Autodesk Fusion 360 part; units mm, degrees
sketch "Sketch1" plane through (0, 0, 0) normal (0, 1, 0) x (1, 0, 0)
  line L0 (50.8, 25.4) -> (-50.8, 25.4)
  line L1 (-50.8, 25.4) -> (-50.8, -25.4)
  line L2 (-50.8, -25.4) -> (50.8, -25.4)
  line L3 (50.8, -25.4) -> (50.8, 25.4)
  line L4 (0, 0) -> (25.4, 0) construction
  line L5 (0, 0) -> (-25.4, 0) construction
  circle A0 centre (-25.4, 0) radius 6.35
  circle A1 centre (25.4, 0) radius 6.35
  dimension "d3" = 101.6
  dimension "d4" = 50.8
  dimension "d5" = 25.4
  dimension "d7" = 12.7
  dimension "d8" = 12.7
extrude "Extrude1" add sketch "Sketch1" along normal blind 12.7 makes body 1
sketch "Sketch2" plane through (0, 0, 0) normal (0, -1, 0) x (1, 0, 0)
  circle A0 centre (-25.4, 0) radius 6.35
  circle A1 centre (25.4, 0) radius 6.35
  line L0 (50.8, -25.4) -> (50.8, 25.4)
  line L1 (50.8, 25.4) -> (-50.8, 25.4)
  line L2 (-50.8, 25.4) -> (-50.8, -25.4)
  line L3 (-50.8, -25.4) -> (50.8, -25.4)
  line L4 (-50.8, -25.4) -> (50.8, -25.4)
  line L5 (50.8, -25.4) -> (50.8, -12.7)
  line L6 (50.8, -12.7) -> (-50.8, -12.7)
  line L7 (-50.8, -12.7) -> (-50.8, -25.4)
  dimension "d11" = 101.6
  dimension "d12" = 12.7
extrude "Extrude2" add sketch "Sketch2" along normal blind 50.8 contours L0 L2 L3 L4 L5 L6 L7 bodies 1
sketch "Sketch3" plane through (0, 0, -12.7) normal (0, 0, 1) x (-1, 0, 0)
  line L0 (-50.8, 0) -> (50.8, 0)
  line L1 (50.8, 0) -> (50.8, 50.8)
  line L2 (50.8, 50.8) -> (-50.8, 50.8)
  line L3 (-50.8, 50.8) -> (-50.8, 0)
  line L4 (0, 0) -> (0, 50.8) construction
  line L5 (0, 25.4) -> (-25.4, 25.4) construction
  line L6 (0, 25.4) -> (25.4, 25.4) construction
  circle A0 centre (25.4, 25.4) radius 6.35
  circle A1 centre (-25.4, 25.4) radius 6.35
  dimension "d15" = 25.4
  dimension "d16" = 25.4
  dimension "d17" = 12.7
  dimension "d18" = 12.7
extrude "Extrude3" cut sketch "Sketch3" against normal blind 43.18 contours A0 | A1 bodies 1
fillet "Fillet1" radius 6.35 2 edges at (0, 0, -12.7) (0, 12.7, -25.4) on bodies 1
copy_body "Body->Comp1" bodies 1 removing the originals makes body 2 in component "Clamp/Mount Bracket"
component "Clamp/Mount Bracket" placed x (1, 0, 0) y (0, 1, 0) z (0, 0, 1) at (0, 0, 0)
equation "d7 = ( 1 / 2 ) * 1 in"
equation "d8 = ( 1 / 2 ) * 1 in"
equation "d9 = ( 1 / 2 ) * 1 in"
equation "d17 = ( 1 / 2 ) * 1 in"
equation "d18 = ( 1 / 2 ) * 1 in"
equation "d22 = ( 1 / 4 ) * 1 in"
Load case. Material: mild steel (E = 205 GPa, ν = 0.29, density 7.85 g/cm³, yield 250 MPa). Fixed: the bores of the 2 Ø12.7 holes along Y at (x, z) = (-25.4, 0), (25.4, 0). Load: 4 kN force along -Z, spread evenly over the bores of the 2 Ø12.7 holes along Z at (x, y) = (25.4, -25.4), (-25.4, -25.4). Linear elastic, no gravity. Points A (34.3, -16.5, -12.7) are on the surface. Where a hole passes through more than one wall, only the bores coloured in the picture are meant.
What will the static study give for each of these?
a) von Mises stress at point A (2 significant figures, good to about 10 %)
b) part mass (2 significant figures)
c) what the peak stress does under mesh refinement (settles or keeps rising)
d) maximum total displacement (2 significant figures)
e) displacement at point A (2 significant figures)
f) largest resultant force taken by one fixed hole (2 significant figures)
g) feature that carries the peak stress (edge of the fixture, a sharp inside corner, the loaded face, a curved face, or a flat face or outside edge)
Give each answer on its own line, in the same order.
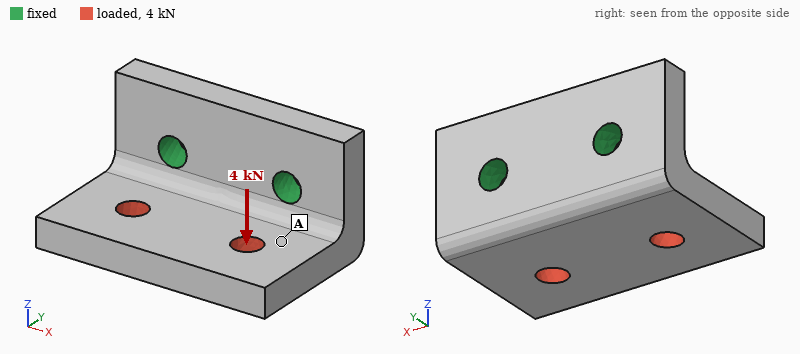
15 MPa
980 g
keeps rising
46 µm
15 µm
2.0 kN
edge of the fixture
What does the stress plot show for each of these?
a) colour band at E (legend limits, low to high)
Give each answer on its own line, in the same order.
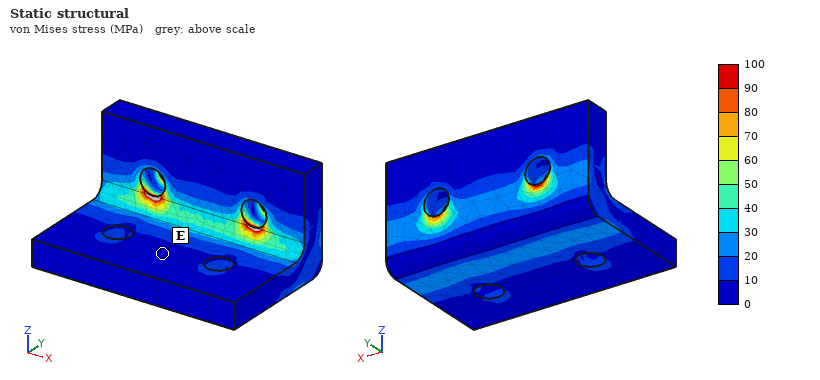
0 to 10 MPa
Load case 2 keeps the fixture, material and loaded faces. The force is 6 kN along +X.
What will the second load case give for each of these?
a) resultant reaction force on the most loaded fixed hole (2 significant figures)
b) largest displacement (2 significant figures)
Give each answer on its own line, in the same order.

4.5 kN
13 µm
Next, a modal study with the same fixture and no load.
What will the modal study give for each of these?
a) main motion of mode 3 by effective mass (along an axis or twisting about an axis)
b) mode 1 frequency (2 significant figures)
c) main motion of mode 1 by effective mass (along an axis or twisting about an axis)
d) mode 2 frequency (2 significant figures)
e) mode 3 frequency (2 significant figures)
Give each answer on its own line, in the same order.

along X
2500 Hz
along Z
4100 Hz
6200 Hz
